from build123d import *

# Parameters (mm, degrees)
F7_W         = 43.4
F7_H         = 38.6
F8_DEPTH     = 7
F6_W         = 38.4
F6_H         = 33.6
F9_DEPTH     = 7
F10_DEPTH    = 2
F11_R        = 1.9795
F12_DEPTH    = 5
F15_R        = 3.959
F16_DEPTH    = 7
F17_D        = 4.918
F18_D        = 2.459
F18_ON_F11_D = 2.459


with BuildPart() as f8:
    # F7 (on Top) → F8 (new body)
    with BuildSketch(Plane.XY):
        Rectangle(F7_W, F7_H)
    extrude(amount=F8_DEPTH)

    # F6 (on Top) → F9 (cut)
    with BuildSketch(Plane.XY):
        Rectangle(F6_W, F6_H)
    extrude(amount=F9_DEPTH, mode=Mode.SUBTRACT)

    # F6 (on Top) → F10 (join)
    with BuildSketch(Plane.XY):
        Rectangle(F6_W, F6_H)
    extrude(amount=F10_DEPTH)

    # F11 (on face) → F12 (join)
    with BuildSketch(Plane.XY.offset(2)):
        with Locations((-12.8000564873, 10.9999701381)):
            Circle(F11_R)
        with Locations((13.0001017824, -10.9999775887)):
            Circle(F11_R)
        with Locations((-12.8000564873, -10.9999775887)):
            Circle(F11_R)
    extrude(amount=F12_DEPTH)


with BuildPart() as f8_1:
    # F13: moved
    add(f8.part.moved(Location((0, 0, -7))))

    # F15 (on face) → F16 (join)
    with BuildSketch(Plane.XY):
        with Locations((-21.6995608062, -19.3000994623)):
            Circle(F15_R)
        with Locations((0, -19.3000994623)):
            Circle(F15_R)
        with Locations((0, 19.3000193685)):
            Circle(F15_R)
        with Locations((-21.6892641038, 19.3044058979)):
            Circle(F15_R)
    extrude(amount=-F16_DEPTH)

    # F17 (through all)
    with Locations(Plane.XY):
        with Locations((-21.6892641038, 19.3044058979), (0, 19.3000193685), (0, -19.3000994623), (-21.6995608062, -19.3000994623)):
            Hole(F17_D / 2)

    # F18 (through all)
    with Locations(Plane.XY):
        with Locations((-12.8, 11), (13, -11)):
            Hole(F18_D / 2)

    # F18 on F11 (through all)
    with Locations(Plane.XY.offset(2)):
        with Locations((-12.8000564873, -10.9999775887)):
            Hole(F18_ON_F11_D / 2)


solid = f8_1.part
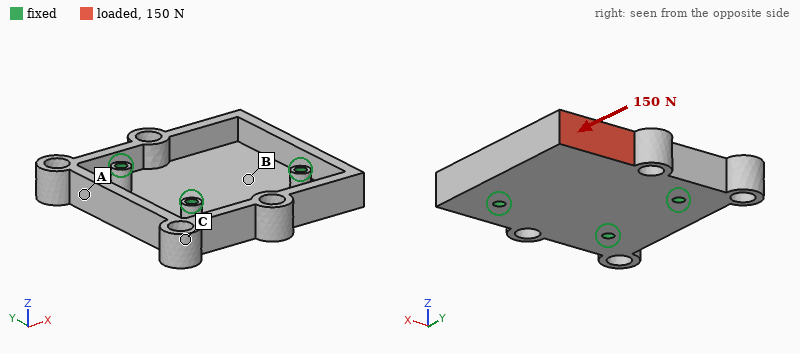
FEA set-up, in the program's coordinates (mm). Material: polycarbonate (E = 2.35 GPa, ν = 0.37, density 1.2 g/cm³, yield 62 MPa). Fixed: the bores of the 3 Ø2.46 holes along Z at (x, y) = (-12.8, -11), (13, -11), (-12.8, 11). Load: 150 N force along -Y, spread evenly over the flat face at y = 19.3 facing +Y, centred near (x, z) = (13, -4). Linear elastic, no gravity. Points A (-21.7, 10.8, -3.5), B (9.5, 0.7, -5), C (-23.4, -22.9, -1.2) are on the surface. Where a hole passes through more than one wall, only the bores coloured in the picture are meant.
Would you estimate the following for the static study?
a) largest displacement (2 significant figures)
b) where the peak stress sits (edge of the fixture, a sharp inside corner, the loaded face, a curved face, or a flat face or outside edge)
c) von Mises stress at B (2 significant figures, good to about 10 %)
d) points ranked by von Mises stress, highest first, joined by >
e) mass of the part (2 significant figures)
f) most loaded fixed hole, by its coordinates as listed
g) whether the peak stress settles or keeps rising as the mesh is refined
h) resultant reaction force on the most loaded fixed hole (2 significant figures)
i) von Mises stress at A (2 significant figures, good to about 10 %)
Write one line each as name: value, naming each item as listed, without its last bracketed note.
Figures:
largest displacement: 0.63 mm
where the peak stress sits: edge of the fixture
von Mises stress at B: 4.6 MPa
points ranked by von Mises stress, highest first, joined by >: B > A > C
mass of the part: 6.9 g
most loaded fixed hole, by its coordinates as listed: (13, -11)
whether the peak stress settles or keeps rising as the mesh is refined: keeps rising
resultant reaction force on the most loaded fixed hole: 120 N
von Mises stress at A: 2.5 MPa
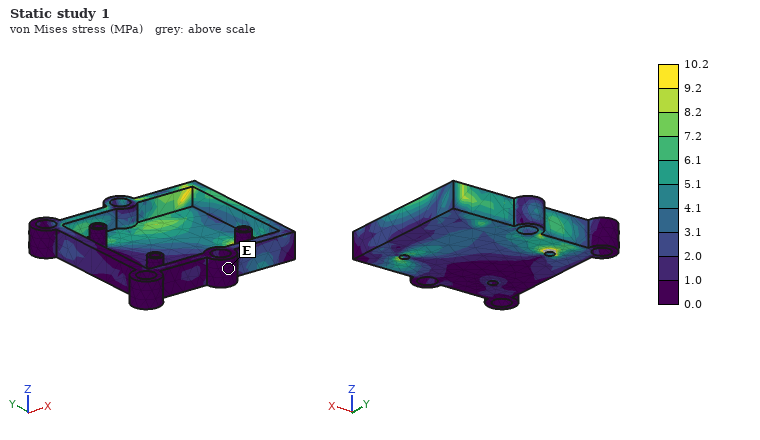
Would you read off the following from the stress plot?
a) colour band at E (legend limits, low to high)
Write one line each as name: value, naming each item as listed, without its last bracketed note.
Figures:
colour band at E: 0.0 to 1.0 MPa
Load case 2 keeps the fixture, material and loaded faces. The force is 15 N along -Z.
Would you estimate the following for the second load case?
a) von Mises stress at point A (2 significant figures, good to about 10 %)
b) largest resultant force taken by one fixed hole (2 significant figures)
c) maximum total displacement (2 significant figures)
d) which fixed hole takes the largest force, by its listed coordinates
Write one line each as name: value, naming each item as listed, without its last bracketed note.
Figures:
von Mises stress at point A: 2.7 MPa
largest resultant force taken by one fixed hole: 14 N
maximum total displacement: 0.70 mm
which fixed hole takes the largest force, by its listed coordinates: (-12.8, 11)
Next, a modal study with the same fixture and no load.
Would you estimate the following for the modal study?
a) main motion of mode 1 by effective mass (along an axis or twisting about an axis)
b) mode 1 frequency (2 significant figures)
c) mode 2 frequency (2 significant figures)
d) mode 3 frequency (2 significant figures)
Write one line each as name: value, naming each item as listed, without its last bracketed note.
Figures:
main motion of mode 1 by effective mass: along Z
mode 1 frequency: 850 Hz
mode 2 frequency: 2900 Hz
mode 3 frequency: 2900 Hz
